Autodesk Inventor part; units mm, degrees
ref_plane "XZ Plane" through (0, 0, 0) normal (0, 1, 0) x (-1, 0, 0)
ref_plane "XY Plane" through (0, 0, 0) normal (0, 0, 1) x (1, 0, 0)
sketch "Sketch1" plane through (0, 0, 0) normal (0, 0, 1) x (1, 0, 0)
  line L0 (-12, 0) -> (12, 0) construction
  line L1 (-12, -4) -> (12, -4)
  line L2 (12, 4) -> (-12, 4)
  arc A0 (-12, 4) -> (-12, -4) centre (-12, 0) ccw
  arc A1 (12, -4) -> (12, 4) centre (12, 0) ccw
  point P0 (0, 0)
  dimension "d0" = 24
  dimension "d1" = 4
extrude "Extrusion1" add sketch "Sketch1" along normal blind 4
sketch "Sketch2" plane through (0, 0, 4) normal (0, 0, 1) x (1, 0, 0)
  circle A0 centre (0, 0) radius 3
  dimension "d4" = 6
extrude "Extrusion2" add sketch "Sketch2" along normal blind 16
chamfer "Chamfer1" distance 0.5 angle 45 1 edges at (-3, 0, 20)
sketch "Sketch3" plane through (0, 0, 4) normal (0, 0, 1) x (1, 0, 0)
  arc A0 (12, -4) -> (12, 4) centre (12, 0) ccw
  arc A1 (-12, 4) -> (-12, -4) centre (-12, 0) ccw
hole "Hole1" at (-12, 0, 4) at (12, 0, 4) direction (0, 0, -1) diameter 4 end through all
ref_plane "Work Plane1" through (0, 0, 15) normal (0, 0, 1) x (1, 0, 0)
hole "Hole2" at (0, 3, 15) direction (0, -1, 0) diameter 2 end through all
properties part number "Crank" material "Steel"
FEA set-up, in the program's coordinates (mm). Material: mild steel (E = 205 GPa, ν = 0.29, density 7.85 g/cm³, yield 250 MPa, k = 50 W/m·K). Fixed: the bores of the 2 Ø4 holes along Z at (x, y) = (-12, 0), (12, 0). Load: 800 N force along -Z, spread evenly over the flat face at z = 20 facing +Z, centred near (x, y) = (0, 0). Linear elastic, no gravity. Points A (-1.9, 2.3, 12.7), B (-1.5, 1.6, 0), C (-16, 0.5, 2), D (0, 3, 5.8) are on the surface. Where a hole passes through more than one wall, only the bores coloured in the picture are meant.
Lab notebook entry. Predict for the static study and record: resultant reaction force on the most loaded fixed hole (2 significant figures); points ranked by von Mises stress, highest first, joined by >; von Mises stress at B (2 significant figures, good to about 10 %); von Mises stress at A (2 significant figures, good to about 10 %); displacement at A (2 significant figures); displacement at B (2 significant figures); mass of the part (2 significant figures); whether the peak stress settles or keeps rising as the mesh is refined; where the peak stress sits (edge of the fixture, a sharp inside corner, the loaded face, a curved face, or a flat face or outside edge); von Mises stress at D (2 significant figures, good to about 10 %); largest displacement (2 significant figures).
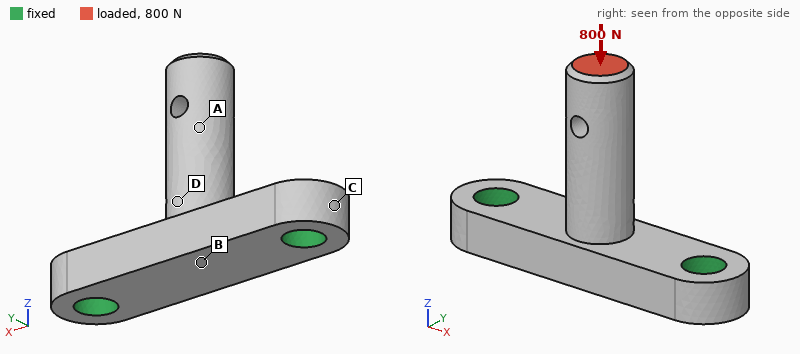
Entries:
410 N
B > A > D > C
56 MPa
39 MPa
6.3 µm
4.9 µm
10 g
keeps rising
edge of the fixture
20 MPa
7.8 µm
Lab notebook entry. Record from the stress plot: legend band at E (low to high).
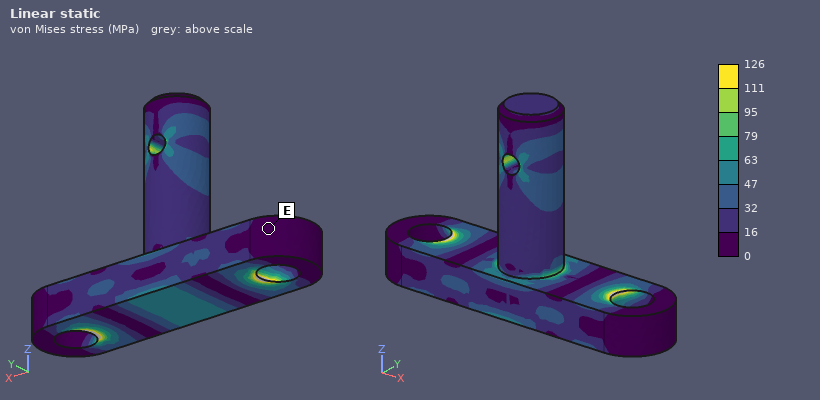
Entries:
0 to 16 MPa
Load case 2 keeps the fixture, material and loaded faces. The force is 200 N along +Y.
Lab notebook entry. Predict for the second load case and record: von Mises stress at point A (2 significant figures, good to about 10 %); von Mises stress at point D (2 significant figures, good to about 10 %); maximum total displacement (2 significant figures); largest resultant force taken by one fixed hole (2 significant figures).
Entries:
71 MPa
130 MPa
58 µm
100 N
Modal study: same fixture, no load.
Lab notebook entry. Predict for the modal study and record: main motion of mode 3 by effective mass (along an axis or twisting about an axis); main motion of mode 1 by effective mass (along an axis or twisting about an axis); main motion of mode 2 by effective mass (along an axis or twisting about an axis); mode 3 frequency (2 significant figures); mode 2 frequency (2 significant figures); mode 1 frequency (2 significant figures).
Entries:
along Z
along Y
along X
25 kHz
12 kHz
9000 Hz
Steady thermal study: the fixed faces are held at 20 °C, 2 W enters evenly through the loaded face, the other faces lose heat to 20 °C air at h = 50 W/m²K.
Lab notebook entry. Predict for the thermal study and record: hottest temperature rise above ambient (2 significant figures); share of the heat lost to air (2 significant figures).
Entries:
29 K
17 %
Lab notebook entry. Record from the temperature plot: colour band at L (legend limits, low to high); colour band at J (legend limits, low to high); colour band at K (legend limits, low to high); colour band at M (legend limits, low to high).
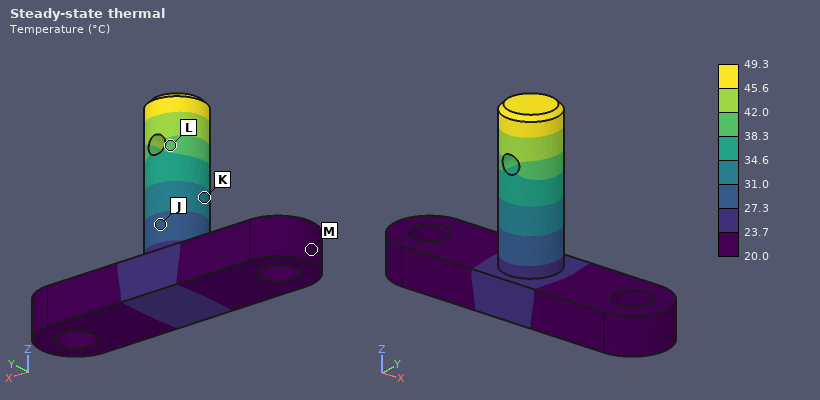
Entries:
38.3 to 42.0 °C
27.3 to 31.0 °C
31.0 to 34.6 °C
20.0 to 23.7 °C
